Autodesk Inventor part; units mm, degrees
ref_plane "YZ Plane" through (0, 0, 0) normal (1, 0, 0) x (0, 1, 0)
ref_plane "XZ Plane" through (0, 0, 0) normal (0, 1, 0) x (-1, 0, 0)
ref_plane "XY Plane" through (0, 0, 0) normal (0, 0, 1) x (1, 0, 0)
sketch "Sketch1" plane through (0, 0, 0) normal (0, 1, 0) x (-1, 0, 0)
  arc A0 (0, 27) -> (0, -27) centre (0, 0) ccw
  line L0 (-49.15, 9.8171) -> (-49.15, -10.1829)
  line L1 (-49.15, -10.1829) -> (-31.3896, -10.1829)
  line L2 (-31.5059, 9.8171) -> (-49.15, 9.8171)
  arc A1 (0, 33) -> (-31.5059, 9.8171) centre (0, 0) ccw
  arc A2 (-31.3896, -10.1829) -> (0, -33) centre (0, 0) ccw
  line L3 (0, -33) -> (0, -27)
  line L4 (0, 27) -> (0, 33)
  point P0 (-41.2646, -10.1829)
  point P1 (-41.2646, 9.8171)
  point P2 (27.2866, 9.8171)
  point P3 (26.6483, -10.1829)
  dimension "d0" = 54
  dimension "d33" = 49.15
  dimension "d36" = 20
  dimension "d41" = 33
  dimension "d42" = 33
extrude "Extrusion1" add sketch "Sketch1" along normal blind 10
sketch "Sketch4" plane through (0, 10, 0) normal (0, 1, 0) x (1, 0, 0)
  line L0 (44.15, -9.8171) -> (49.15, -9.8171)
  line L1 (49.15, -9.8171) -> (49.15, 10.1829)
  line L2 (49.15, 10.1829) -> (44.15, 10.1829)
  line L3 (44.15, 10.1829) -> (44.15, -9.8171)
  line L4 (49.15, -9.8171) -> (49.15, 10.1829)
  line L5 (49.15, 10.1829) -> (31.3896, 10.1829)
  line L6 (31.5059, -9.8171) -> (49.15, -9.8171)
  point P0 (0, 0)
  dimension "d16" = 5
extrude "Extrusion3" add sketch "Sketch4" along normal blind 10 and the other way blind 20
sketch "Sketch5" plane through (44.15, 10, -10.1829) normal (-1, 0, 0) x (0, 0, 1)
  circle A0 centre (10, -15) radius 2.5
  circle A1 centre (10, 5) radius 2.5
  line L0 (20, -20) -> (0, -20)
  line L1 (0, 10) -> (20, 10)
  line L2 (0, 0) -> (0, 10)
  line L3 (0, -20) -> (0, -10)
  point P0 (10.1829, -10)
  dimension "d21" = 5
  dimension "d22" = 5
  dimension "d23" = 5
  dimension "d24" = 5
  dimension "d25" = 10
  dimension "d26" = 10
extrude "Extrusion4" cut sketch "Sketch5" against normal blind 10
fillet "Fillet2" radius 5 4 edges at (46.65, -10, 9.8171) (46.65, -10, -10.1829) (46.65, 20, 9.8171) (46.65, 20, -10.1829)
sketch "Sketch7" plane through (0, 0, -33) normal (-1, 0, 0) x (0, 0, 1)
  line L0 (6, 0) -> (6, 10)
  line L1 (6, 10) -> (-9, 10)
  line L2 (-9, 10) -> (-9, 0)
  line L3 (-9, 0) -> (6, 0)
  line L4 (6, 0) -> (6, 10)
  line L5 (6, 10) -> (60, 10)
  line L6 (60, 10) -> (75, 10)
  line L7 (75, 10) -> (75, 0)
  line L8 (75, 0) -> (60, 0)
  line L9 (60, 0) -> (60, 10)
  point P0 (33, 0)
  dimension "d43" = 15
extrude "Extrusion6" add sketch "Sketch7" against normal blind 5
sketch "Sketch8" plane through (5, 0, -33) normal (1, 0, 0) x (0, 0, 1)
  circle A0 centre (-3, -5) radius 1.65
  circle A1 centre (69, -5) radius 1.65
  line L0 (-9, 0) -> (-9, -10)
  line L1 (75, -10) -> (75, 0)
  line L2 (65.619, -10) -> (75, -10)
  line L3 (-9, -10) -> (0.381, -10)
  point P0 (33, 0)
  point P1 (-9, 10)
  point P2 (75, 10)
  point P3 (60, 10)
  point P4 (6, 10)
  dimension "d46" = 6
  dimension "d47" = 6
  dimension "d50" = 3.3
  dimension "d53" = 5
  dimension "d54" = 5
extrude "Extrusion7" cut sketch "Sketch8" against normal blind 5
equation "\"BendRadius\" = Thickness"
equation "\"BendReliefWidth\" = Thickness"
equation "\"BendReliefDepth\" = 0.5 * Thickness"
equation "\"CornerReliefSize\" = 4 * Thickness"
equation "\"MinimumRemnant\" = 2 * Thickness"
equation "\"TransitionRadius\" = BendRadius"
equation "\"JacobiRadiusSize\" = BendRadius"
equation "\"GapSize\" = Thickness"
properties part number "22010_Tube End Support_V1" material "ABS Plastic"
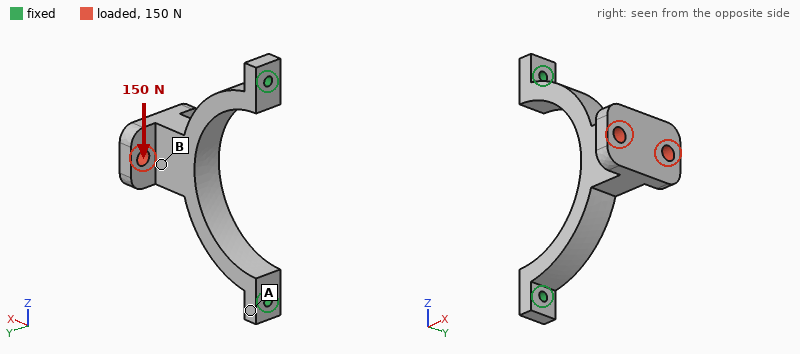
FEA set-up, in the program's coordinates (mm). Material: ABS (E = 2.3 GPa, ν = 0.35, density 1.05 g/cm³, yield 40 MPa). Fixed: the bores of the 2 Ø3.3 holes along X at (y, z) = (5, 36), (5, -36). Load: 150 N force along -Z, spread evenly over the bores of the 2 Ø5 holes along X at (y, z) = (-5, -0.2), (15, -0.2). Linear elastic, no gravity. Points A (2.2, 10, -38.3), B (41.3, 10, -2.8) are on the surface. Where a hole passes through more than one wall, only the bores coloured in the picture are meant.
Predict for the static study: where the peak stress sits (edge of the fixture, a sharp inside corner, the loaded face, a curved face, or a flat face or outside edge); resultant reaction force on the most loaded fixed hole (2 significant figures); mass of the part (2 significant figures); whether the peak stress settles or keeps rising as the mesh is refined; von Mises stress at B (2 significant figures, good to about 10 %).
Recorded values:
edge of the fixture
120 N
12 g
keeps rising
2.1 MPa
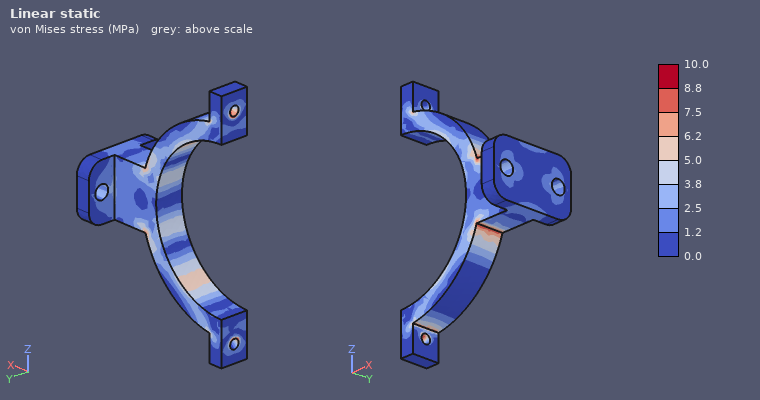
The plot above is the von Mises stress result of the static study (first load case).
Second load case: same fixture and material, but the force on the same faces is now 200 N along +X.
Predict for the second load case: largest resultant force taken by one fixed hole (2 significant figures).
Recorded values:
130 N
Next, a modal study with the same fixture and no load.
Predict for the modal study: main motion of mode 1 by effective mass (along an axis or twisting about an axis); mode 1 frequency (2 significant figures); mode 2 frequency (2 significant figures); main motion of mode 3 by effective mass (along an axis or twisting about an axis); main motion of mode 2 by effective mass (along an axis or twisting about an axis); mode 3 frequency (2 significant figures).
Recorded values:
along Y
370 Hz
1600 Hz
twisting about X
along Z
2000 Hz
